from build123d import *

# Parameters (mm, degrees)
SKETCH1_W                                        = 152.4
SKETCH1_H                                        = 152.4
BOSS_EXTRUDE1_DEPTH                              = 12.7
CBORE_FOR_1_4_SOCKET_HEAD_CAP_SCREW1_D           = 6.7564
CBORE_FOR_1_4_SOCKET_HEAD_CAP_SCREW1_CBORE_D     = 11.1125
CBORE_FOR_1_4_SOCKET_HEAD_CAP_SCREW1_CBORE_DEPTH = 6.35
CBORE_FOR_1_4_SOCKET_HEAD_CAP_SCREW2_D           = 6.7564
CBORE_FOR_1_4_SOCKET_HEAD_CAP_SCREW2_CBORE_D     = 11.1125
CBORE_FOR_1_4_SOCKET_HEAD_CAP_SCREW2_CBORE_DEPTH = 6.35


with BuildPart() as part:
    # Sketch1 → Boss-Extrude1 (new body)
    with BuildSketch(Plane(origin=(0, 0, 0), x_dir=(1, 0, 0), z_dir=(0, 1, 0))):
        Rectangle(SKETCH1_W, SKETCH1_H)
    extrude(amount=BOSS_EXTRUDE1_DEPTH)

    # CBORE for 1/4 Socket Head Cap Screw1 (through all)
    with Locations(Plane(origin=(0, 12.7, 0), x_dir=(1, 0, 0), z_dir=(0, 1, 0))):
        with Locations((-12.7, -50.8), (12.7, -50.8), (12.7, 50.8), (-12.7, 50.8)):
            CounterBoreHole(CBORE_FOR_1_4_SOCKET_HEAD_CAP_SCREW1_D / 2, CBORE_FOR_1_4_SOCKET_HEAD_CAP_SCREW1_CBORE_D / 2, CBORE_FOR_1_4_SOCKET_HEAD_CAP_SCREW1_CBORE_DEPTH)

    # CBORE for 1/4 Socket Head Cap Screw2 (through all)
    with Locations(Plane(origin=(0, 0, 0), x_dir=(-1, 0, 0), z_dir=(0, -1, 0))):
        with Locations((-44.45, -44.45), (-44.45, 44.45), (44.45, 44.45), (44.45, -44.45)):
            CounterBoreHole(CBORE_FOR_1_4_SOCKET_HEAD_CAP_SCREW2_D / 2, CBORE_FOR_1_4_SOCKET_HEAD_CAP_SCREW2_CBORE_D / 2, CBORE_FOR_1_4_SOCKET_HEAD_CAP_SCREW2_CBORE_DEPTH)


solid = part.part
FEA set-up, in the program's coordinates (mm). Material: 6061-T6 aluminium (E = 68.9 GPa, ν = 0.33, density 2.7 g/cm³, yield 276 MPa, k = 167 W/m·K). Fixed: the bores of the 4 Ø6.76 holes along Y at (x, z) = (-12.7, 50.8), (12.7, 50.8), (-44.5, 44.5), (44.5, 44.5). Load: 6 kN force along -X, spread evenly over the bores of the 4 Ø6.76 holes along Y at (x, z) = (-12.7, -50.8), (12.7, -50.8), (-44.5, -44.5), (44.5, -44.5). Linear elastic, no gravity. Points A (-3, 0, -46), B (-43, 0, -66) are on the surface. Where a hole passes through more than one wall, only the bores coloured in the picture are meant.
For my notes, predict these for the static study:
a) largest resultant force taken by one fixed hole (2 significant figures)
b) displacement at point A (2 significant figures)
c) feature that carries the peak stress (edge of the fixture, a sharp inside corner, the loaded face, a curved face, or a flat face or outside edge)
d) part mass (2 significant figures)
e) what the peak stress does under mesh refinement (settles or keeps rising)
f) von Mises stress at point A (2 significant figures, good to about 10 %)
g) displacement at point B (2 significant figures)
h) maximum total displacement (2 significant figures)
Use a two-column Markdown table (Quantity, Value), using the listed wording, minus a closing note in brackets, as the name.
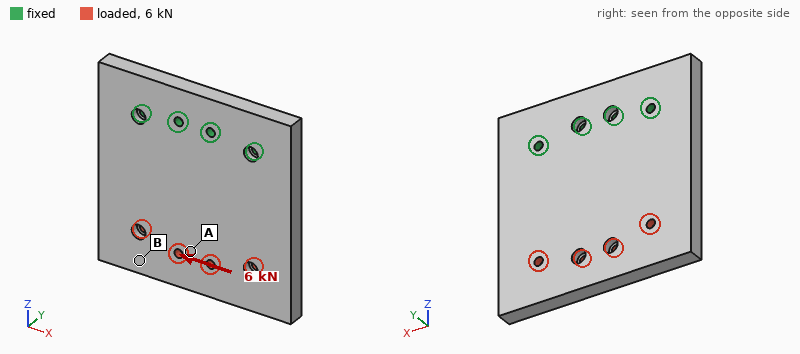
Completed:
| Quantity | Value |
|---|---|
| largest resultant force taken by one fixed hole | 6.1 kN |
| displacement at point A | 32 µm |
| feature that carries the peak stress | edge of the fixture |
| part mass | 780 g |
| what the peak stress does under mesh refinement | keeps rising |
| von Mises stress at point A | 10 MPa |
| displacement at point B | 40 µm |
| maximum total displacement | 51 µm |
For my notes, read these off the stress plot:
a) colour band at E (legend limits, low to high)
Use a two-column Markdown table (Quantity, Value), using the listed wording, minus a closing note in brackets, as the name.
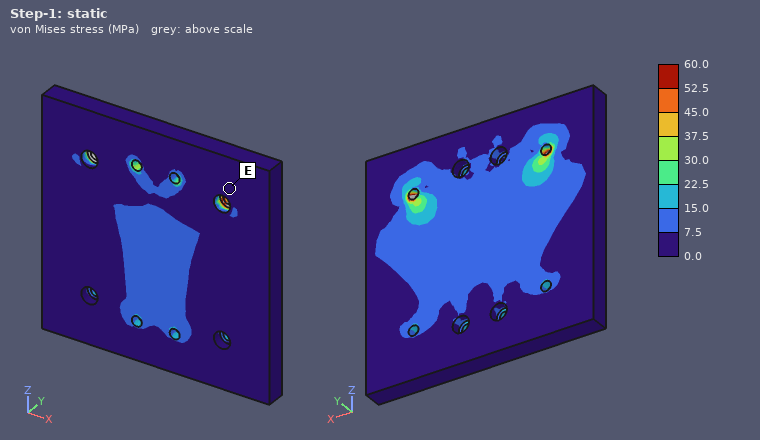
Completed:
| Quantity | Value |
|---|---|
| colour band at E | 0.0 to 7.5 MPa |
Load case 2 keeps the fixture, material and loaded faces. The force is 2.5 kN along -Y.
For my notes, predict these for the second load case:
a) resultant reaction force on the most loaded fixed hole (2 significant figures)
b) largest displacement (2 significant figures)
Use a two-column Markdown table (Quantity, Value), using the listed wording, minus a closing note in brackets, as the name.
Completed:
| Quantity | Value |
|---|---|
| resultant reaction force on the most loaded fixed hole | 5.9 kN |
| largest displacement | 0.83 mm |
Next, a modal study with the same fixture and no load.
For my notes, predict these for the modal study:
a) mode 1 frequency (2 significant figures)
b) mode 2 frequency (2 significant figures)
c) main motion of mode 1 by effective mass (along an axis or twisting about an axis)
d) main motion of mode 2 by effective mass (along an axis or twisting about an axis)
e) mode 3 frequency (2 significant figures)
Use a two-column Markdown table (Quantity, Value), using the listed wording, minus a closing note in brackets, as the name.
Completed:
| Quantity | Value |
|---|---|
| mode 1 frequency | 570 Hz |
| mode 2 frequency | 1200 Hz |
| main motion of mode 1 by effective mass | along Y |
| main motion of mode 2 by effective mass | twisting about Z |
| mode 3 frequency | 3200 Hz |
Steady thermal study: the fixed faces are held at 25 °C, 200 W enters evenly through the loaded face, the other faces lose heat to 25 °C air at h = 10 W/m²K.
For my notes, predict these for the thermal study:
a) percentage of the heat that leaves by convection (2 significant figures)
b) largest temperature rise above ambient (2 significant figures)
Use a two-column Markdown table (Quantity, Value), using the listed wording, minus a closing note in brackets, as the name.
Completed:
| Quantity | Value |
|---|---|
| percentage of the heat that leaves by convection | 9.2 % |
| largest temperature rise above ambient | 73 K |
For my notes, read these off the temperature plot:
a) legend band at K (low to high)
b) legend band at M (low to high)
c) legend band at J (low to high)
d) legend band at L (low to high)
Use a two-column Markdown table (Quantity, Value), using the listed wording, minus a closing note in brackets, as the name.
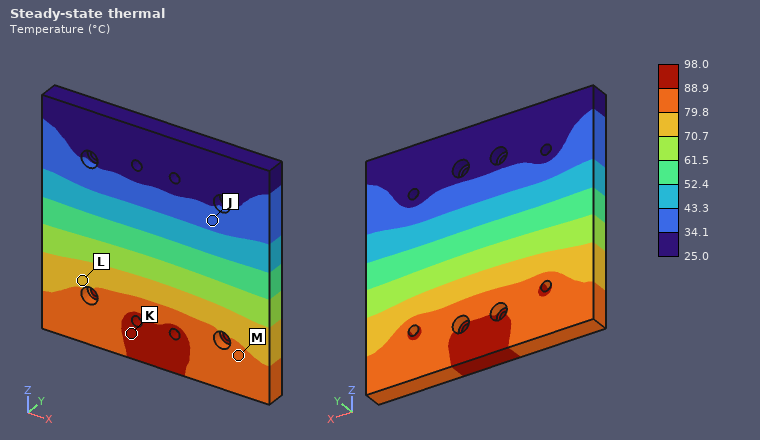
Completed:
| Quantity | Value |
|---|---|
| legend band at K | 88.9 to 98.0 °C |
| legend band at M | 79.8 to 88.9 °C |
| legend band at J | 34.1 to 43.3 °C |
| legend band at L | 70.7 to 79.8 °C |
